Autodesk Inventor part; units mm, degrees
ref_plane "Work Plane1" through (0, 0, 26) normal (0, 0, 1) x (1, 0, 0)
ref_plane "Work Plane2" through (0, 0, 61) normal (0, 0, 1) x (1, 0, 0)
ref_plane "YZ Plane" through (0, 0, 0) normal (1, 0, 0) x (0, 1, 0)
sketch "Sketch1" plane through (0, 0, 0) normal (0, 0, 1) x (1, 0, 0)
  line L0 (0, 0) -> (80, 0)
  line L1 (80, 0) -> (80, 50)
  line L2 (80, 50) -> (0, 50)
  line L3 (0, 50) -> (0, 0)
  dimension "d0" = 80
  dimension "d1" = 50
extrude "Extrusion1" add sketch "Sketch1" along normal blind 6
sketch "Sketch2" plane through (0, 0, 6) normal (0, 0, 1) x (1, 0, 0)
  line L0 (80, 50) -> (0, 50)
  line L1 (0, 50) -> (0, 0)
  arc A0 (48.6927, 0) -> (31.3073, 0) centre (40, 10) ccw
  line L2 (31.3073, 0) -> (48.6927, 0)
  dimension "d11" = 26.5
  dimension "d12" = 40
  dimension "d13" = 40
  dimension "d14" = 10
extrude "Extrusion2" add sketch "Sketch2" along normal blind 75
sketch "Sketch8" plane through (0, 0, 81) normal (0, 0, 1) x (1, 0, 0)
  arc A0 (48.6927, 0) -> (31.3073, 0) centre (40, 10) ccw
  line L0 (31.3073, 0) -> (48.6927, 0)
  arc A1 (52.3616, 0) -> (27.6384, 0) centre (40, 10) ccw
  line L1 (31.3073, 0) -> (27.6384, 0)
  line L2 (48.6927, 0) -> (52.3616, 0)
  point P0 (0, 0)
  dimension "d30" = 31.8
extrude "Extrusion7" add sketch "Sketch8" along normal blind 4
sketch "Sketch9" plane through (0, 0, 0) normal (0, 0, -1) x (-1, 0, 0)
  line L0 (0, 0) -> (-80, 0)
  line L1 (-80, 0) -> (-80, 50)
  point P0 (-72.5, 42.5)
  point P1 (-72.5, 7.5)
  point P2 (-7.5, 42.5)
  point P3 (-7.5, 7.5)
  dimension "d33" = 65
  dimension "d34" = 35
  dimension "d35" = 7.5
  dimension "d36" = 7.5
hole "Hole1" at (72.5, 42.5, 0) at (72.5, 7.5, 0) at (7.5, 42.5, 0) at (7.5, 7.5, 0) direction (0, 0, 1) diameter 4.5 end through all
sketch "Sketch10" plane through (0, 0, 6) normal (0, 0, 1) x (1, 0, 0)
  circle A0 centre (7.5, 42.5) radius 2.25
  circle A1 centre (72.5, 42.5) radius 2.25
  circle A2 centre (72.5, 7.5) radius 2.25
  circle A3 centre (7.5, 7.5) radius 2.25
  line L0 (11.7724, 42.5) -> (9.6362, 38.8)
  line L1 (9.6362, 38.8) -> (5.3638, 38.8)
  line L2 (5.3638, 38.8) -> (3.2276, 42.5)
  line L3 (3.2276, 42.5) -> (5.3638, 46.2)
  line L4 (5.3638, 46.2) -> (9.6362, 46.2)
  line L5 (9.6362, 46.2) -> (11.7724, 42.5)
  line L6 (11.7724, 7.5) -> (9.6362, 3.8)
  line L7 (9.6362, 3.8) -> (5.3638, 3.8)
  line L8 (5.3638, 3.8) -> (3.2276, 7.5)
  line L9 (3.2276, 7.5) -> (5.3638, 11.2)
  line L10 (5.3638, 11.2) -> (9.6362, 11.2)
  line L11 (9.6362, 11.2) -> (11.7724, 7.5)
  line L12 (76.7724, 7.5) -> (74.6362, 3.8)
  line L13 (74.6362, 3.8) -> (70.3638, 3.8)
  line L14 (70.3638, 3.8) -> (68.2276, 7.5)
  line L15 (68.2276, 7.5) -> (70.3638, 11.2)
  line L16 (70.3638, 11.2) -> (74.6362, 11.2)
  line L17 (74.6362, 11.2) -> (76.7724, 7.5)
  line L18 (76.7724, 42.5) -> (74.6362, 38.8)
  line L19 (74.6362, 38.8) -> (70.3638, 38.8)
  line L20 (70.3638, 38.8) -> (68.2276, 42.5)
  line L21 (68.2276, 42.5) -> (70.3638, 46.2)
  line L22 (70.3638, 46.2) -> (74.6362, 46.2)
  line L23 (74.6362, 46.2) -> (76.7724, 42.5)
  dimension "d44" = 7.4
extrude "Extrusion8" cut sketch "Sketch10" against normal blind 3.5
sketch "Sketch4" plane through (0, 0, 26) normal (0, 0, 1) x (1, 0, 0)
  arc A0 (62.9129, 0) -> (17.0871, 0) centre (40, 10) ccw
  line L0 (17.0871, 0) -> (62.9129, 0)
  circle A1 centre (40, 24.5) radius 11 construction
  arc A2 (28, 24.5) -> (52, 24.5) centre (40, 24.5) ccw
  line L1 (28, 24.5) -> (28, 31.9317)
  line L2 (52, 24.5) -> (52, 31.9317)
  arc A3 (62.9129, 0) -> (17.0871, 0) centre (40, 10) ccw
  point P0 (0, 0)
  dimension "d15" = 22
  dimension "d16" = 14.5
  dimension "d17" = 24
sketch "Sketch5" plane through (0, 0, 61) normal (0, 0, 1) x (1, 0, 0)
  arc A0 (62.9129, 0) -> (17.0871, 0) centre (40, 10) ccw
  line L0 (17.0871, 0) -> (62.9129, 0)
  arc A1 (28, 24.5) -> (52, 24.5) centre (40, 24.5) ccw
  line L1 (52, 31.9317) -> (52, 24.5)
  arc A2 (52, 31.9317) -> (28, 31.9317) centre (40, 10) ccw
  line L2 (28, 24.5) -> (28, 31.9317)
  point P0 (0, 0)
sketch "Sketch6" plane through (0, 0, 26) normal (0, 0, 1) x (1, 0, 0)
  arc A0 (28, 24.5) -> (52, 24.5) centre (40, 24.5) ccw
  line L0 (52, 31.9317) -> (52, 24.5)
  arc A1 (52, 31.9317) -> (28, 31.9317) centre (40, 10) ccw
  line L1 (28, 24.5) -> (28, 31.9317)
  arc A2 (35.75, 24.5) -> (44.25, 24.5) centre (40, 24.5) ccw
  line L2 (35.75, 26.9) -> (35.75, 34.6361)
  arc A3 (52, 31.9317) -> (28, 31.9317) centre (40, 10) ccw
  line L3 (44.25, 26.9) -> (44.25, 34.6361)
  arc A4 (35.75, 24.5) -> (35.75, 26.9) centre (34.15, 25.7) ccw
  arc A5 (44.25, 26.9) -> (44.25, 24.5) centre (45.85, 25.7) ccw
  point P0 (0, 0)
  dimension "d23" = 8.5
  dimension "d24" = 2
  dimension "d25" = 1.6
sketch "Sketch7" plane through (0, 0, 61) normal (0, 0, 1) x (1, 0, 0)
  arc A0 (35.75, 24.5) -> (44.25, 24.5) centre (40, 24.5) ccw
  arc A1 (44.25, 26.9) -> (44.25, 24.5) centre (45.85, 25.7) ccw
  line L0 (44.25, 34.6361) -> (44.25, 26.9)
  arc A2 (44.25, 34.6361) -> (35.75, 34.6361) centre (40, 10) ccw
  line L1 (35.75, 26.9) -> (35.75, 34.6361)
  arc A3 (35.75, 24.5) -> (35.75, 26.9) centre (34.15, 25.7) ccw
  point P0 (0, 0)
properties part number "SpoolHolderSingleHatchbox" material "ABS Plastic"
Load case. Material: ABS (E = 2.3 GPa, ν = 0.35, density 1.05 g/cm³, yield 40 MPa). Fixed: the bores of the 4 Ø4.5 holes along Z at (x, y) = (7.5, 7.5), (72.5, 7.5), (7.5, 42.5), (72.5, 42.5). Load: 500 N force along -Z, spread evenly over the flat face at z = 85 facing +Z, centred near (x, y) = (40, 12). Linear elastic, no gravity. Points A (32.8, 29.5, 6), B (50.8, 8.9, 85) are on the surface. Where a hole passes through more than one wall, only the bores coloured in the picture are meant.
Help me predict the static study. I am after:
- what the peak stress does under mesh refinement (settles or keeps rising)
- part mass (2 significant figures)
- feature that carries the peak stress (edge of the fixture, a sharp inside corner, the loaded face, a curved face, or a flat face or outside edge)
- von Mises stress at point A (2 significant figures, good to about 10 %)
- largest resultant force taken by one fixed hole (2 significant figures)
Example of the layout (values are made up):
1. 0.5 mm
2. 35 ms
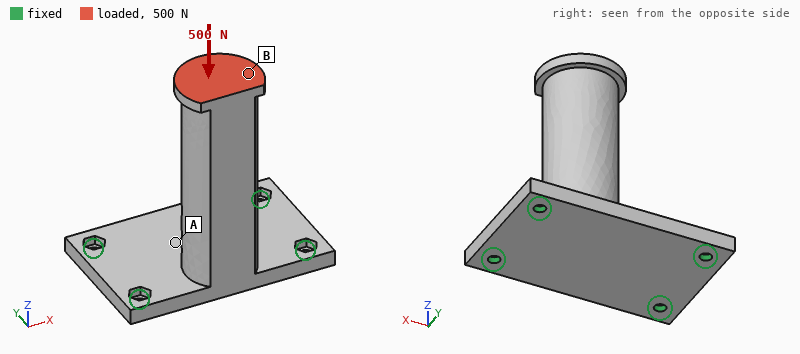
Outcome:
1. keeps rising
2. 68 g
3. edge of the fixture
4. 4.6 MPa
5. 370 N
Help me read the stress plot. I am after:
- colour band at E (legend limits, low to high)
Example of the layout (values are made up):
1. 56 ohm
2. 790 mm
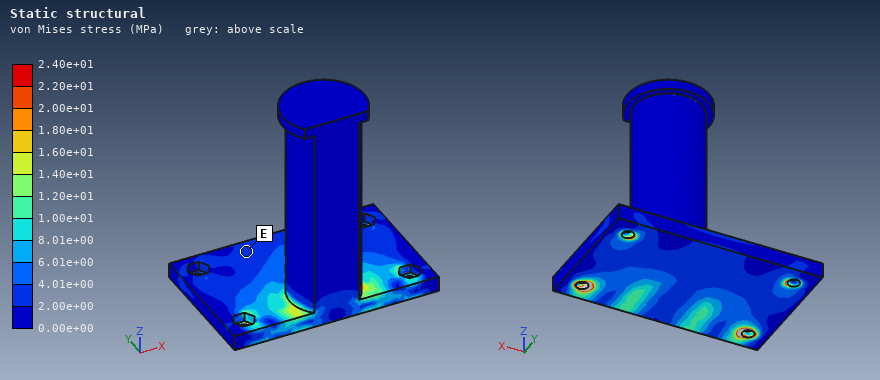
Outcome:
1. 2.00e+00 to 4.01e+00 MPa
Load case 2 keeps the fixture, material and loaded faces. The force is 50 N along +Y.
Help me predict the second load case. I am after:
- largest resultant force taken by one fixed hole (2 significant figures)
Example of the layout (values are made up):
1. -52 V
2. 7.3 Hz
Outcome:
1. 96 N
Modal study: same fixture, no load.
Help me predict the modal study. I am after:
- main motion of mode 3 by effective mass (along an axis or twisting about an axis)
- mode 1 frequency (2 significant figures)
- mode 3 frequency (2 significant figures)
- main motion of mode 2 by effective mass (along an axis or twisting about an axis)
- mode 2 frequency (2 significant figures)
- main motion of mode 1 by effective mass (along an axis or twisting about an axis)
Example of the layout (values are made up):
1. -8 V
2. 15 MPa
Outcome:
1. along Z
2. 250 Hz
3. 800 Hz
4. along X
5. 390 Hz
6. along Y
